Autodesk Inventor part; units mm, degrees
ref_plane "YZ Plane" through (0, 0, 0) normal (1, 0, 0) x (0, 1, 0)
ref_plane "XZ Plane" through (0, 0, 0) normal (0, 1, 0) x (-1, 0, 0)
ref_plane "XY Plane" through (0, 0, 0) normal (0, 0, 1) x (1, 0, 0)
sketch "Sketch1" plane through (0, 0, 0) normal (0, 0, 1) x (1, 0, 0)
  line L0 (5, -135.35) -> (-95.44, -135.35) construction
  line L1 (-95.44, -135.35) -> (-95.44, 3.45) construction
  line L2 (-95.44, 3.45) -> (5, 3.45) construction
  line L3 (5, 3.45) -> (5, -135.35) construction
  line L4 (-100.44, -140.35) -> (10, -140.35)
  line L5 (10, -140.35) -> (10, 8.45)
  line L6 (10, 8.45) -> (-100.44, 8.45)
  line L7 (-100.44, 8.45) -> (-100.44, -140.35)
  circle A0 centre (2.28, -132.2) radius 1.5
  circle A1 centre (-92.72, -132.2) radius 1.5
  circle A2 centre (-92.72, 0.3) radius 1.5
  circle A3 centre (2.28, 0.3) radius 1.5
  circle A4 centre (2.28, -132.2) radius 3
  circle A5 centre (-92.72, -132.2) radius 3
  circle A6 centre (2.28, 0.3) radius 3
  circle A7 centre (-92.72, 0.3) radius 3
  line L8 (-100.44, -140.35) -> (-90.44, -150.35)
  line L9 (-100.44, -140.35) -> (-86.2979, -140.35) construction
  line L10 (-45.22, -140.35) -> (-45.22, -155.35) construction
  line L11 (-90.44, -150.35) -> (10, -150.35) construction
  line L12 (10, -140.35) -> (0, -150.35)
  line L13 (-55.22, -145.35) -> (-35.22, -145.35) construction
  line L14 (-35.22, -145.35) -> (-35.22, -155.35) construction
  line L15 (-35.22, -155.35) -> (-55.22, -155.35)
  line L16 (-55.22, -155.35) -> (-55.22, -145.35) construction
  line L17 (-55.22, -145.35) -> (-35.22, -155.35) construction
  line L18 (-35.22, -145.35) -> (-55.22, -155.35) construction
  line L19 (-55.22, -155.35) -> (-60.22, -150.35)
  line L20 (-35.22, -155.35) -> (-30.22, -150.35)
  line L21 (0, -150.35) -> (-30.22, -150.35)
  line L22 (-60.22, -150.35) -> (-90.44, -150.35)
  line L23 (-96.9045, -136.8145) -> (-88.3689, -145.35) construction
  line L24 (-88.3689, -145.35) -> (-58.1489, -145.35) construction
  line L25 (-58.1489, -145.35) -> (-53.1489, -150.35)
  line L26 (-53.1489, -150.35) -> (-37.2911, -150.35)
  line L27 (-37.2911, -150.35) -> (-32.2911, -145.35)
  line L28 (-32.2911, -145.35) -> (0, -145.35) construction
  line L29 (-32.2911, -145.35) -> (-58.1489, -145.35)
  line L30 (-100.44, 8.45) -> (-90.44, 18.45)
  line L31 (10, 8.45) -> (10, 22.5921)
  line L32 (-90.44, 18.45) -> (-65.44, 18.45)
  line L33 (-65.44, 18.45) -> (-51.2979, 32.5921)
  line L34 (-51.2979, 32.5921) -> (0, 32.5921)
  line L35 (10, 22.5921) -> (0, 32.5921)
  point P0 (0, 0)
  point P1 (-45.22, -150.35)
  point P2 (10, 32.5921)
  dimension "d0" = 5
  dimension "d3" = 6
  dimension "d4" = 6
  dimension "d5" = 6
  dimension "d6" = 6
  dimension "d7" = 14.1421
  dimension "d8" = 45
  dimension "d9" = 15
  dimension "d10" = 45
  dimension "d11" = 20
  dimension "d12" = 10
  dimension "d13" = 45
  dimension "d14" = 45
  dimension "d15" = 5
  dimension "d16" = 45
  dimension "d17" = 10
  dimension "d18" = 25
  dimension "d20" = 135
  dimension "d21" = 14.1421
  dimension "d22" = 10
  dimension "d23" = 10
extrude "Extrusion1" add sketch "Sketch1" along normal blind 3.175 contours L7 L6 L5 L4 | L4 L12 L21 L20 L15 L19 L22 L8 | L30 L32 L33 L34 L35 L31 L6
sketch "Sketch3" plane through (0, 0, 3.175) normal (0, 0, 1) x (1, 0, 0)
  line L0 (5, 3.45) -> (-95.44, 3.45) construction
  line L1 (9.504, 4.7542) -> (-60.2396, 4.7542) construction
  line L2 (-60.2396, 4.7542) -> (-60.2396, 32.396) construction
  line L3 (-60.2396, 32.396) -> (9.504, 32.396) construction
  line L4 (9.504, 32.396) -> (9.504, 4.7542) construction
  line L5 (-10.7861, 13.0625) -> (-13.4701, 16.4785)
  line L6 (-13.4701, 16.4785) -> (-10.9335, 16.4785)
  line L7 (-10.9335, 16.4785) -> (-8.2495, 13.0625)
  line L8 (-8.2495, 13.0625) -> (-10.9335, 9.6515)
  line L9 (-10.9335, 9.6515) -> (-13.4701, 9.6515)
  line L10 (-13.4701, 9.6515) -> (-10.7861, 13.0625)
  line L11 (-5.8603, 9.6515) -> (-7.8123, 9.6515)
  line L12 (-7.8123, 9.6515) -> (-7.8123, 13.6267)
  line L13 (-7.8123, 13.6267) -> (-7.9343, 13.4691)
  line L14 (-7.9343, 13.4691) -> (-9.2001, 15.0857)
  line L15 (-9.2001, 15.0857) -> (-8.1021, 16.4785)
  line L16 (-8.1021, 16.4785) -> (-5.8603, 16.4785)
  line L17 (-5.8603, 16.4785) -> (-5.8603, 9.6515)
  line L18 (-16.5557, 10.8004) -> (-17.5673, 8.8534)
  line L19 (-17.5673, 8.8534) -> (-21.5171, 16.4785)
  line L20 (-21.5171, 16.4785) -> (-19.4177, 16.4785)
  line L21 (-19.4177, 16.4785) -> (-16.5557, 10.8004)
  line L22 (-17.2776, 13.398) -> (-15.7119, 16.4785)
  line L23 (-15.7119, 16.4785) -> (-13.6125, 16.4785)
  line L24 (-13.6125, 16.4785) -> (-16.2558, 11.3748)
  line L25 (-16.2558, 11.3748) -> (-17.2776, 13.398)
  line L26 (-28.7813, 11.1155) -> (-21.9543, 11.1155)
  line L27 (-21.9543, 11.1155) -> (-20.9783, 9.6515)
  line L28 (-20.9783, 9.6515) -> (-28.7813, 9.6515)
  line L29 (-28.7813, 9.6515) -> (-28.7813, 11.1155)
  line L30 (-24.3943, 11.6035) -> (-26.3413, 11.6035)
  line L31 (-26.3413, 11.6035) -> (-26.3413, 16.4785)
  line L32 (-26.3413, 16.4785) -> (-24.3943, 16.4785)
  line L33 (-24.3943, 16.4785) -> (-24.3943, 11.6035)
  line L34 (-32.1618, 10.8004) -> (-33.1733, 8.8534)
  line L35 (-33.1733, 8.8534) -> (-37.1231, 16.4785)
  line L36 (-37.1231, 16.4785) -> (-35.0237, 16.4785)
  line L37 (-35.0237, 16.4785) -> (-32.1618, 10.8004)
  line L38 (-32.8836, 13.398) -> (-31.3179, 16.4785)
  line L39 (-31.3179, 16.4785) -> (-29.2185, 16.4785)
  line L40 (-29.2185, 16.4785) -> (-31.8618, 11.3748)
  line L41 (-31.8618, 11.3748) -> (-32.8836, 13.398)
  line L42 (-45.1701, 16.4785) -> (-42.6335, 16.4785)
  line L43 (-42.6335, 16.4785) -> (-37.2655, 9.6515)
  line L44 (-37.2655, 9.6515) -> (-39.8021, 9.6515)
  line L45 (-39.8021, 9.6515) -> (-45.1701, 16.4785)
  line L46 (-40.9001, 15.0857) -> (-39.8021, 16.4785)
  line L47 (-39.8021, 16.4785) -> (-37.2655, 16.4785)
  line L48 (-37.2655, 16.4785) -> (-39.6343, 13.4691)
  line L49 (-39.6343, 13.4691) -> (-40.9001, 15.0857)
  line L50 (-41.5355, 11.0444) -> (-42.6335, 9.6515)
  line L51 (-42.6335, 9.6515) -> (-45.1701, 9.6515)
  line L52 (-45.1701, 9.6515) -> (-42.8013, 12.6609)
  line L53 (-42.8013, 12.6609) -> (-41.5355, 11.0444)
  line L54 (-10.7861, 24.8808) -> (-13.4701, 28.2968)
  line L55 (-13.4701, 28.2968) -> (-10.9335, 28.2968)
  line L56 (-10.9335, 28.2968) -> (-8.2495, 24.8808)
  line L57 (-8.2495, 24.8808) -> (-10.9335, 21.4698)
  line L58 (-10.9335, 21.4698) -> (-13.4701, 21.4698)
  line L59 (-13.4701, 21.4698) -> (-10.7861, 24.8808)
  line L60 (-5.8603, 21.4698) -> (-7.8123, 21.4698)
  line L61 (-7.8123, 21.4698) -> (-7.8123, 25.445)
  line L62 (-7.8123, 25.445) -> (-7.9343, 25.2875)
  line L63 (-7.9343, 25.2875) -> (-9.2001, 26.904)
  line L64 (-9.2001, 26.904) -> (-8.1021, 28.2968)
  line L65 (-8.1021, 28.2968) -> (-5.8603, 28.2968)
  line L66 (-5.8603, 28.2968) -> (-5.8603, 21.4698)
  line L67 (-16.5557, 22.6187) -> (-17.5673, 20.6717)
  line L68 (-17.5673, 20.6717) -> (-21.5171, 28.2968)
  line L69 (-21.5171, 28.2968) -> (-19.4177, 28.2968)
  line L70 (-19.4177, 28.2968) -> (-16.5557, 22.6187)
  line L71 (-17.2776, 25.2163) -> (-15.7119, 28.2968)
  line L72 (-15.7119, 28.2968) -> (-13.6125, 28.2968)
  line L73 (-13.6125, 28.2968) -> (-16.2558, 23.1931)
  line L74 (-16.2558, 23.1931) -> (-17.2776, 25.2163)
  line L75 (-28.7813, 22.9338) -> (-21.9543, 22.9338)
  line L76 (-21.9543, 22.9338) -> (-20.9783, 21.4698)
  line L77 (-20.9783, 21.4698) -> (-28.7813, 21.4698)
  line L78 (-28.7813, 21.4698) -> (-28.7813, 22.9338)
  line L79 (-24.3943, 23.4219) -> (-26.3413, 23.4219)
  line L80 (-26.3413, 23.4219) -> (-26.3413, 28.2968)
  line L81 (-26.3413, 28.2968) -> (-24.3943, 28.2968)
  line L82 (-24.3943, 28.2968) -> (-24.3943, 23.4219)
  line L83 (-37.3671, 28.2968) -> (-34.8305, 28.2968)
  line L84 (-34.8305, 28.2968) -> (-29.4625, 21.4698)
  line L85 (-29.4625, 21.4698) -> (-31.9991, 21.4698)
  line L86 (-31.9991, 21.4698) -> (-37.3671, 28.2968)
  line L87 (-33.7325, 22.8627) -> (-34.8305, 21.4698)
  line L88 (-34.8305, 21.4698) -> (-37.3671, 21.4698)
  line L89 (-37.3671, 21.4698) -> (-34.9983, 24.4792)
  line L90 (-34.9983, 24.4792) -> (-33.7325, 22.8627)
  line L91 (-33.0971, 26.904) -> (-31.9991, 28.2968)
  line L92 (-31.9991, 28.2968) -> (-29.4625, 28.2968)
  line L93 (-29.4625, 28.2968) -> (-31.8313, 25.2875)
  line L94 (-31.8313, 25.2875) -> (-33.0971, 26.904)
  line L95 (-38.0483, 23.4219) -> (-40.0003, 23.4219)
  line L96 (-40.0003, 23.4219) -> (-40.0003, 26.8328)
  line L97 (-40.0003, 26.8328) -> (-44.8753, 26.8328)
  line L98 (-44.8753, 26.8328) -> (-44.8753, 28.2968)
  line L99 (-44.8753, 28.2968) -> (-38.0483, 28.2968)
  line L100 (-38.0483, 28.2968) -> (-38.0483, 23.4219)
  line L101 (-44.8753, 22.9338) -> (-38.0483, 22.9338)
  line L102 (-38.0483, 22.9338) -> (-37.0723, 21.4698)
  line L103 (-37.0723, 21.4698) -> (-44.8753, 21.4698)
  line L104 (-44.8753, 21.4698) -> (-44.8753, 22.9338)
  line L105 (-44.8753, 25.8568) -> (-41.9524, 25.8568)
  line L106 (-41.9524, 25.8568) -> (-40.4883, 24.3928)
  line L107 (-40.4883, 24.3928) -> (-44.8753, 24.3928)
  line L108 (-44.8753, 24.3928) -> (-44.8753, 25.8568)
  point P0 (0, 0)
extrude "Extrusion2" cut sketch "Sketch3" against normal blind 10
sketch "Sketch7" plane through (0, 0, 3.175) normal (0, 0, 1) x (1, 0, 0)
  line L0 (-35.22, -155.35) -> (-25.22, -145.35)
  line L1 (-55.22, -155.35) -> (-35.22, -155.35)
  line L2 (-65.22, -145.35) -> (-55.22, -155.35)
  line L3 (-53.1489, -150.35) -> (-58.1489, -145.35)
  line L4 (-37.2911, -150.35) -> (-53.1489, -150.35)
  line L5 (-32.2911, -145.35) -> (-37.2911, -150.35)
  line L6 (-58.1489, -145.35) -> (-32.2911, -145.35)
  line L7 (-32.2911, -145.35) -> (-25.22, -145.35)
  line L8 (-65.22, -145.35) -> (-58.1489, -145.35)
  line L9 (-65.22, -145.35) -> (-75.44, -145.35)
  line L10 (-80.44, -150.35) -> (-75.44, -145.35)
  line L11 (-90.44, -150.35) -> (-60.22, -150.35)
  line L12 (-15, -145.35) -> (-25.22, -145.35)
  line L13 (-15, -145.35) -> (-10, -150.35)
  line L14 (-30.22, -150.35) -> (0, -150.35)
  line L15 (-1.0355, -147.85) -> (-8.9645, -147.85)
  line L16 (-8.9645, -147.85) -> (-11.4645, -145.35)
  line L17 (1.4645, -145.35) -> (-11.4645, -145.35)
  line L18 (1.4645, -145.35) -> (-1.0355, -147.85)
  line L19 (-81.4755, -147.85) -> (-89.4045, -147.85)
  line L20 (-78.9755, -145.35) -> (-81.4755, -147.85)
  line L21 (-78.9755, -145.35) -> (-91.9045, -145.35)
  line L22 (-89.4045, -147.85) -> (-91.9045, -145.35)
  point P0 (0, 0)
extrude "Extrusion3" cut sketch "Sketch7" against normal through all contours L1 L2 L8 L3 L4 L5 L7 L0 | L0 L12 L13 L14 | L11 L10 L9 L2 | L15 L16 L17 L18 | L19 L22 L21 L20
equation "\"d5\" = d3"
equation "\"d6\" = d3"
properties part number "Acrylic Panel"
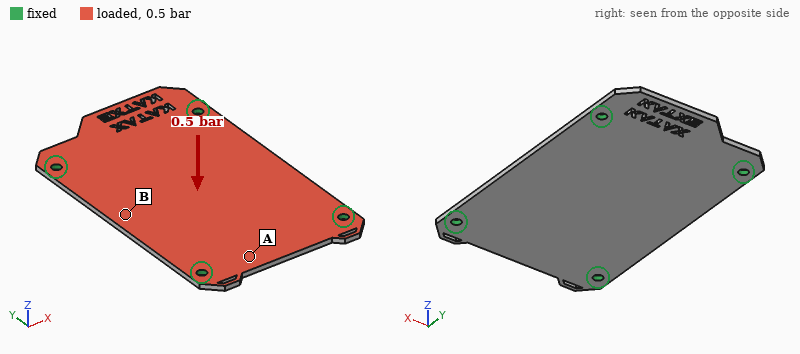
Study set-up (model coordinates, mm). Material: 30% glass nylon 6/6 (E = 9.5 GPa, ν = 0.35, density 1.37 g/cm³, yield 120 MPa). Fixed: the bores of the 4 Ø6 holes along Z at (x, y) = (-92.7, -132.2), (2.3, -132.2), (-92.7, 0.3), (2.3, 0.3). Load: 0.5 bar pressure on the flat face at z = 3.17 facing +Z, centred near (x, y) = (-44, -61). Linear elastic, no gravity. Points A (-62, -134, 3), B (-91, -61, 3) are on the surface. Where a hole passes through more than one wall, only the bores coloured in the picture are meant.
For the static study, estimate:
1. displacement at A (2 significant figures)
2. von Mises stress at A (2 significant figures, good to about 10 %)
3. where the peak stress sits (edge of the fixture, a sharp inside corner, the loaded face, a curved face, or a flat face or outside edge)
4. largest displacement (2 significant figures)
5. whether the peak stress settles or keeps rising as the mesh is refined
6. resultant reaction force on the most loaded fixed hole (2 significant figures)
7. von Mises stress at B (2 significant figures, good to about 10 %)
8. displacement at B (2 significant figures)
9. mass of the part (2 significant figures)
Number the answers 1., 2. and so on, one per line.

1. 0.41 mm
2. 12 MPa
3. edge of the fixture
4. 2.4 mm
5. keeps rising
6. 260 N
7. 26 MPa
8. 2.0 mm
9. 81 g
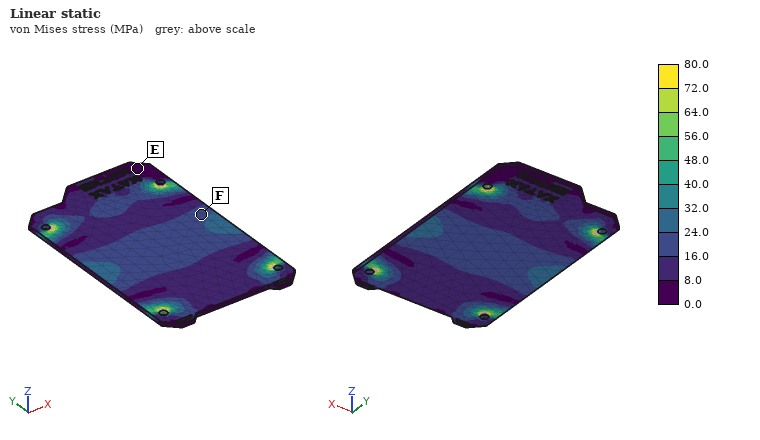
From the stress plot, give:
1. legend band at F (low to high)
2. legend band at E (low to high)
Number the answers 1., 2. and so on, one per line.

1. 16.0 to 24.0 MPa
2. 0.0 to 8.0 MPa
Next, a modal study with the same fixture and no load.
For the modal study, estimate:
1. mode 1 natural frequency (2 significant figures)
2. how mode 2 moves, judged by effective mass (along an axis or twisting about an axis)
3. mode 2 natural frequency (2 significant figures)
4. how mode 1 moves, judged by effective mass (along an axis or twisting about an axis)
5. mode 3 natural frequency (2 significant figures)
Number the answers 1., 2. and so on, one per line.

1. 410 Hz
2. twisting about Y
3. 640 Hz
4. along Z
5. 800 Hz
